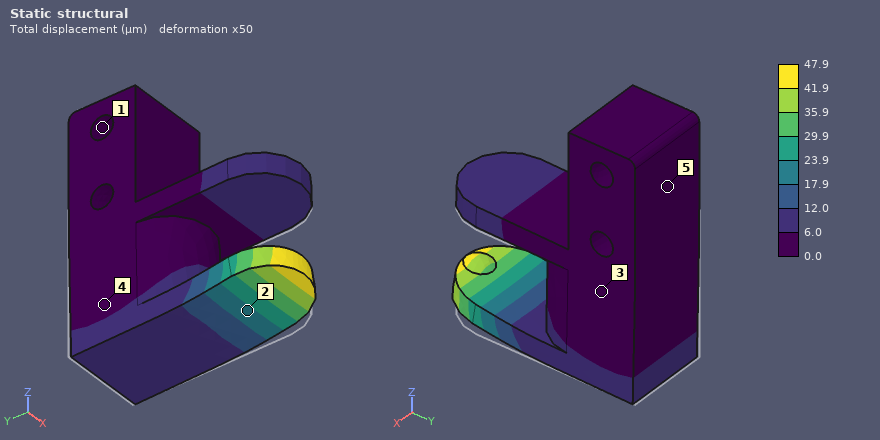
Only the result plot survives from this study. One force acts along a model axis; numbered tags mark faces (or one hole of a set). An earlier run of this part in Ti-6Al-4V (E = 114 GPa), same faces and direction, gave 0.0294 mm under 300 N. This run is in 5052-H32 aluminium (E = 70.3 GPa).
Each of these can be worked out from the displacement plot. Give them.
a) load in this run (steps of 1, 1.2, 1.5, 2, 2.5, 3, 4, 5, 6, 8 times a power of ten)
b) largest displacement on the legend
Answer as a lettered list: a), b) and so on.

a) 300 N
b) 47.9 µm
